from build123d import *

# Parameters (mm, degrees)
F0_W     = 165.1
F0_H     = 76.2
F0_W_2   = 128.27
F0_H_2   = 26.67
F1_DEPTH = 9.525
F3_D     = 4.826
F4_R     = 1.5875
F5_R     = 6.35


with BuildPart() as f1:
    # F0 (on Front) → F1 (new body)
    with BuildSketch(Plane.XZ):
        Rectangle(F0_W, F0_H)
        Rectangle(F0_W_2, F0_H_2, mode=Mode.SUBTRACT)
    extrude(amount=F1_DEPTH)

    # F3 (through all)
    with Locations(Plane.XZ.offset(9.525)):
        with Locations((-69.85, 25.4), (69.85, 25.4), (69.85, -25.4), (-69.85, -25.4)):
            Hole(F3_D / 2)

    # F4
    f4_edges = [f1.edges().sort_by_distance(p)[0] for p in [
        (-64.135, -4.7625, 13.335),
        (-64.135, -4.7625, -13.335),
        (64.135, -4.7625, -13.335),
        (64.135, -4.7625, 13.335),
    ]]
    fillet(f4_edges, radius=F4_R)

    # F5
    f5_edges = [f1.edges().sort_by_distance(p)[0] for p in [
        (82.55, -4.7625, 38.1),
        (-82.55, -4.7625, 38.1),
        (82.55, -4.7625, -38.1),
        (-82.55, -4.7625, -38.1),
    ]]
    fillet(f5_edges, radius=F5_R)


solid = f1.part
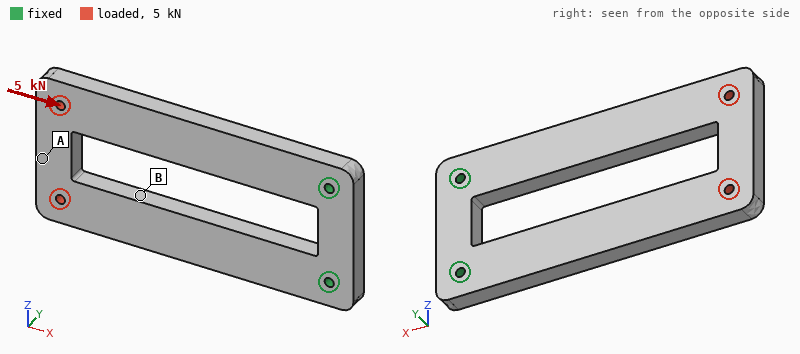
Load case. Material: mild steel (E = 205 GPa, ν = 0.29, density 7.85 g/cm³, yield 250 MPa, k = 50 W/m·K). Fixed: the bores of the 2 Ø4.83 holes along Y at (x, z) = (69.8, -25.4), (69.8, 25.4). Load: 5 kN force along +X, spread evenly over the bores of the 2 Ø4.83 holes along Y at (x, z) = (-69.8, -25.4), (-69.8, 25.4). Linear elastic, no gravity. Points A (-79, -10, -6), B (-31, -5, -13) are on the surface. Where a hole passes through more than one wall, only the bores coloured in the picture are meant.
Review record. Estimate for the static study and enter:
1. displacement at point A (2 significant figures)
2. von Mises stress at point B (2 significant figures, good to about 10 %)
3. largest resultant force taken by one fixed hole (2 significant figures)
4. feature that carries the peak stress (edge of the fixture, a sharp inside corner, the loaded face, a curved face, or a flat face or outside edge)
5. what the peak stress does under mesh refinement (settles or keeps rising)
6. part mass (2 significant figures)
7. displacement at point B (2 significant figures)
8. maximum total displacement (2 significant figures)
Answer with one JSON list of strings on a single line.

["7.5 µm", "12 MPa", "2.5 kN", "edge of the fixture", "keeps rising", "680 g", "5.6 µm", "8.1 µm"]
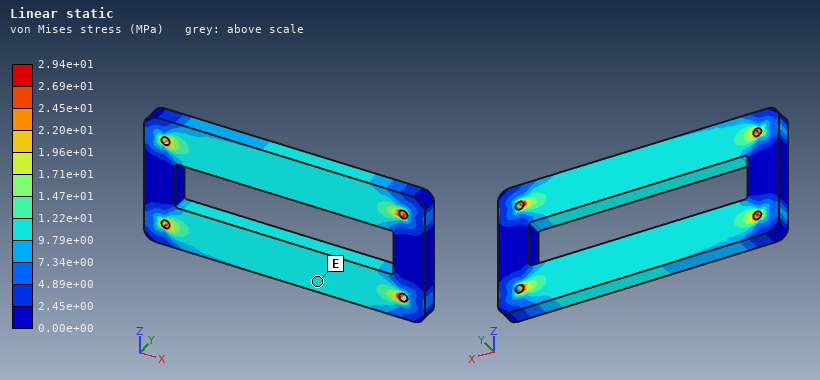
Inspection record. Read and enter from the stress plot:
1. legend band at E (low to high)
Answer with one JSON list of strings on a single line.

["9.79e+00 to 1.22e+01 MPa"]
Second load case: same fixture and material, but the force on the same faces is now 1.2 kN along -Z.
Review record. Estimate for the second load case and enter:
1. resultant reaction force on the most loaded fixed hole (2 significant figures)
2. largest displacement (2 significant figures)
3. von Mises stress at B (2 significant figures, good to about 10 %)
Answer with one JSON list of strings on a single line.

["2.8 kN", "0.11 mm", "22 MPa"]
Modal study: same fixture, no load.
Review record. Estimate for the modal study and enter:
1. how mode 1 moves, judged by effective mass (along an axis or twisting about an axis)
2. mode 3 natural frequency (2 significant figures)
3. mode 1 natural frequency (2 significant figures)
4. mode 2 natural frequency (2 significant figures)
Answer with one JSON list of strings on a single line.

["along Y", "1100 Hz", "300 Hz", "1100 Hz"]
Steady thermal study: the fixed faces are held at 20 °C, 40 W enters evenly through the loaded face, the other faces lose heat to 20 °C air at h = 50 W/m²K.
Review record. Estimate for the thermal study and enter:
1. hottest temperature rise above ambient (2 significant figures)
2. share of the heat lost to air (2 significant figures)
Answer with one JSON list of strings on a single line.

["78 K", "87 %"]
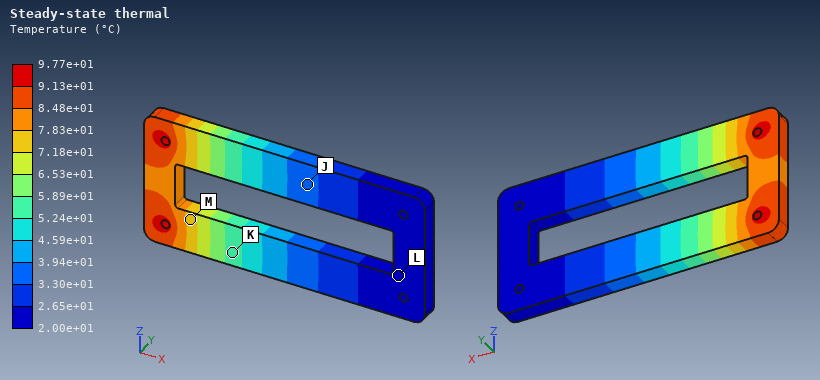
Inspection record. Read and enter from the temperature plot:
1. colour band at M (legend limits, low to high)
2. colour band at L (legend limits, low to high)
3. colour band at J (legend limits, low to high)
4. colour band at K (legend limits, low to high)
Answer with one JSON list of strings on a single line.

["7.18e+01 to 7.83e+01 °C", "2.00e+01 to 2.65e+01 °C", "3.30e+01 to 3.94e+01 °C", "5.24e+01 to 5.89e+01 °C"]
